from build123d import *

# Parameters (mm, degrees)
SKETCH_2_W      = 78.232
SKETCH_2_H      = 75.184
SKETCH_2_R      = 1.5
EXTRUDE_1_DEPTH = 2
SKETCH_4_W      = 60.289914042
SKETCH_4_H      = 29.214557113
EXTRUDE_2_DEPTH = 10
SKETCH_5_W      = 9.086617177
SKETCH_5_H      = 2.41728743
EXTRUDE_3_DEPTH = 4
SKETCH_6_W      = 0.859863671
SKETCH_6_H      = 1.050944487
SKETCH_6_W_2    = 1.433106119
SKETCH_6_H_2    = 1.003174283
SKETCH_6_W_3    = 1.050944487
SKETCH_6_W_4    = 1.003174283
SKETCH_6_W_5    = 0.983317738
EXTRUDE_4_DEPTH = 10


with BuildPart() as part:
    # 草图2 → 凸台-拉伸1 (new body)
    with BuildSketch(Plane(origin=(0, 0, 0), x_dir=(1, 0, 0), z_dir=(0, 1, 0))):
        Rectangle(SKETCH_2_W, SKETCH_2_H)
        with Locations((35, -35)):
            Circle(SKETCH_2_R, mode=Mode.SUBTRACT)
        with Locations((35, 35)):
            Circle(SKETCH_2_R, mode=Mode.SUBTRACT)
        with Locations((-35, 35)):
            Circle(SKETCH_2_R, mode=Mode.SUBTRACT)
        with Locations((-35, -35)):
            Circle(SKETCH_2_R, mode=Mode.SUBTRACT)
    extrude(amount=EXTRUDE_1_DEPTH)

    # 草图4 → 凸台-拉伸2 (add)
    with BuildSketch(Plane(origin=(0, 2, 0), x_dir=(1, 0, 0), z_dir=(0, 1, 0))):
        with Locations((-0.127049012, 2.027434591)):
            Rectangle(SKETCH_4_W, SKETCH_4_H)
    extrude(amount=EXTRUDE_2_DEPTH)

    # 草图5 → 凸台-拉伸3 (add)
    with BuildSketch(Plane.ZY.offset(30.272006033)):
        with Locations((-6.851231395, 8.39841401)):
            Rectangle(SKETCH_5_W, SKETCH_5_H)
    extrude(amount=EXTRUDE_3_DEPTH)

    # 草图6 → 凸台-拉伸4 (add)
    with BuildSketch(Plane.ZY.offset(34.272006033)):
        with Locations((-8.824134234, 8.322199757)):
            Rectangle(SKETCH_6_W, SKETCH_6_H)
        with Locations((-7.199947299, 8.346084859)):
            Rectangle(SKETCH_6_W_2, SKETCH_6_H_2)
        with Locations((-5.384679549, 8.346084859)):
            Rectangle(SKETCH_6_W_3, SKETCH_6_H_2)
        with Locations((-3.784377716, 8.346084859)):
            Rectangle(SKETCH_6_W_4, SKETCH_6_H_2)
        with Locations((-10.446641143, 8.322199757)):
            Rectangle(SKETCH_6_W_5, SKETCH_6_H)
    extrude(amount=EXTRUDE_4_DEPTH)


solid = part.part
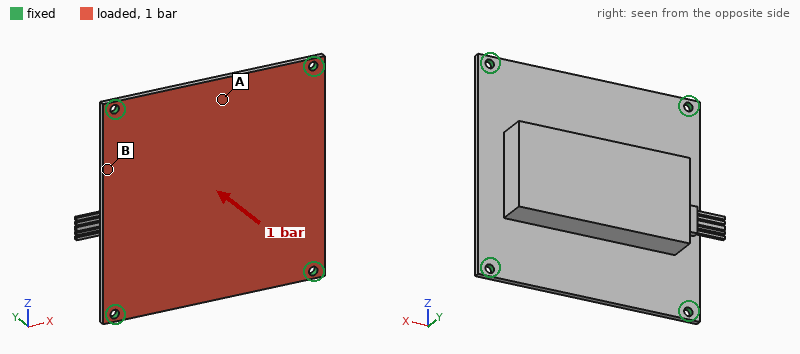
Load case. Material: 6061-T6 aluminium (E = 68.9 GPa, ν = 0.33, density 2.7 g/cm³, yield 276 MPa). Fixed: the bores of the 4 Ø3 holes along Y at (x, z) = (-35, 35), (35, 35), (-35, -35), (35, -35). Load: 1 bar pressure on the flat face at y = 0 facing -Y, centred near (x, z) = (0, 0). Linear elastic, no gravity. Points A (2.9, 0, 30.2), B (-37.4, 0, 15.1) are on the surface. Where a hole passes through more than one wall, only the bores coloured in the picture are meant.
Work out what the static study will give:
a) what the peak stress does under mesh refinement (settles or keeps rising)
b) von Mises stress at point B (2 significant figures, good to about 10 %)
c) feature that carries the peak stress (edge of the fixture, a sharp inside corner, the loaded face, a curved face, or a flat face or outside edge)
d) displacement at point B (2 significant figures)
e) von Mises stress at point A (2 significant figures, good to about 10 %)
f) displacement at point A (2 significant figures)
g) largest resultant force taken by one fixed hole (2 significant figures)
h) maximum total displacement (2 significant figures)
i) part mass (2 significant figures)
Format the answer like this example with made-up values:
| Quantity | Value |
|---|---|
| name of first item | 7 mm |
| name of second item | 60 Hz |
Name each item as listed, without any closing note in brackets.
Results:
| Quantity | Value |
|---|---|
| what the peak stress does under mesh refinement | keeps rising |
| von Mises stress at point B | 48 MPa |
| feature that carries the peak stress | edge of the fixture |
| displacement at point B | 0.11 mm |
| von Mises stress at point A | 20 MPa |
| displacement at point A | 0.14 mm |
| largest resultant force taken by one fixed hole | 150 N |
| maximum total displacement | 0.14 mm |
| part mass | 80 g |
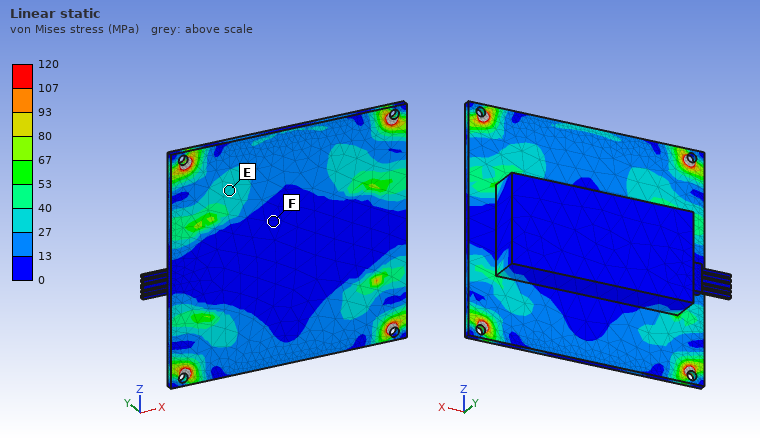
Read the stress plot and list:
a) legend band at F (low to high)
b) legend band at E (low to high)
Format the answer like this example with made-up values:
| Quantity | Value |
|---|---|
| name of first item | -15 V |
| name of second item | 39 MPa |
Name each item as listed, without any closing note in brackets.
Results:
| Quantity | Value |
|---|---|
| legend band at F | 0 to 13 MPa |
| legend band at E | 27 to 40 MPa |
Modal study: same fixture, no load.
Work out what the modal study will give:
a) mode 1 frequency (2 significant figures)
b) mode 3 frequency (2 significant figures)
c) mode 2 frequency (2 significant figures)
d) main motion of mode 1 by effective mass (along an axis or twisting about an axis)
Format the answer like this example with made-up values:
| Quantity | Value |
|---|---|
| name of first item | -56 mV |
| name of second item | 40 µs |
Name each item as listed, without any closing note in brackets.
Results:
| Quantity | Value |
|---|---|
| mode 1 frequency | 1100 Hz |
| mode 3 frequency | 2500 Hz |
| mode 2 frequency | 1900 Hz |
| main motion of mode 1 by effective mass | along Y |
